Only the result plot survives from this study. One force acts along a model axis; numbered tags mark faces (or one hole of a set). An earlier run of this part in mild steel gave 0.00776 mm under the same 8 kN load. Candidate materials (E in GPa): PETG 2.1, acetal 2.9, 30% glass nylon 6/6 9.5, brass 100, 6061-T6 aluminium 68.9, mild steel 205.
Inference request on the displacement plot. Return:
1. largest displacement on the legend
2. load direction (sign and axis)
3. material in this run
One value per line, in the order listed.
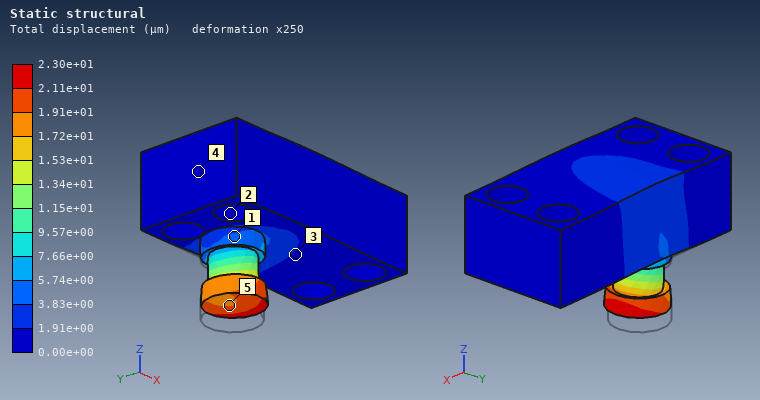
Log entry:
2.30e+01 µm
+Z
6061-T6 aluminium
